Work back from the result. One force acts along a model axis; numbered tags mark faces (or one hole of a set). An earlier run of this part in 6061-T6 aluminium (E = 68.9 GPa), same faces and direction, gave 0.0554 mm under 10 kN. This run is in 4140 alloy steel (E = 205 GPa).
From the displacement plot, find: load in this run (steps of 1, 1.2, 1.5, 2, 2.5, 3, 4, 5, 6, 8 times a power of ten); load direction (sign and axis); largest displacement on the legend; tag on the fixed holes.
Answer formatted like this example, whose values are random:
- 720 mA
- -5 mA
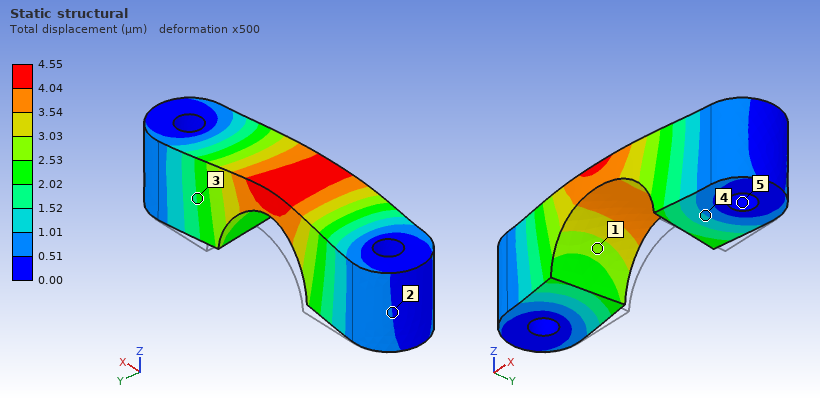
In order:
- 2.5 kN
- -Y
- 4.55 µm
- 5
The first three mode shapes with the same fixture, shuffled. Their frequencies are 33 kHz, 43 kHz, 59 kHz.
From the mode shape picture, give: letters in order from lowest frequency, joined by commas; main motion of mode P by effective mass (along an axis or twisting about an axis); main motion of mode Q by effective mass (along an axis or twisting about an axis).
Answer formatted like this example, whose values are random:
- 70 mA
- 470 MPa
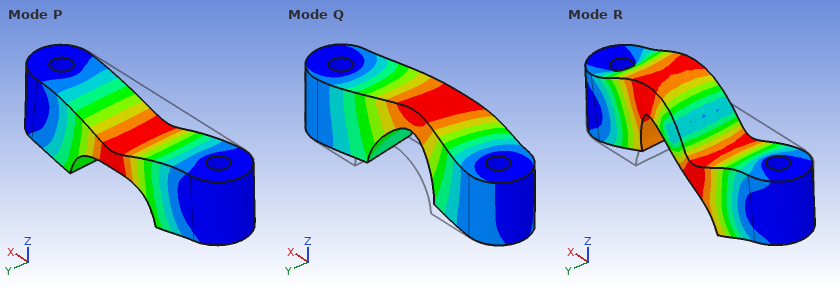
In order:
- Q, P, R
- along Z
- along Y
